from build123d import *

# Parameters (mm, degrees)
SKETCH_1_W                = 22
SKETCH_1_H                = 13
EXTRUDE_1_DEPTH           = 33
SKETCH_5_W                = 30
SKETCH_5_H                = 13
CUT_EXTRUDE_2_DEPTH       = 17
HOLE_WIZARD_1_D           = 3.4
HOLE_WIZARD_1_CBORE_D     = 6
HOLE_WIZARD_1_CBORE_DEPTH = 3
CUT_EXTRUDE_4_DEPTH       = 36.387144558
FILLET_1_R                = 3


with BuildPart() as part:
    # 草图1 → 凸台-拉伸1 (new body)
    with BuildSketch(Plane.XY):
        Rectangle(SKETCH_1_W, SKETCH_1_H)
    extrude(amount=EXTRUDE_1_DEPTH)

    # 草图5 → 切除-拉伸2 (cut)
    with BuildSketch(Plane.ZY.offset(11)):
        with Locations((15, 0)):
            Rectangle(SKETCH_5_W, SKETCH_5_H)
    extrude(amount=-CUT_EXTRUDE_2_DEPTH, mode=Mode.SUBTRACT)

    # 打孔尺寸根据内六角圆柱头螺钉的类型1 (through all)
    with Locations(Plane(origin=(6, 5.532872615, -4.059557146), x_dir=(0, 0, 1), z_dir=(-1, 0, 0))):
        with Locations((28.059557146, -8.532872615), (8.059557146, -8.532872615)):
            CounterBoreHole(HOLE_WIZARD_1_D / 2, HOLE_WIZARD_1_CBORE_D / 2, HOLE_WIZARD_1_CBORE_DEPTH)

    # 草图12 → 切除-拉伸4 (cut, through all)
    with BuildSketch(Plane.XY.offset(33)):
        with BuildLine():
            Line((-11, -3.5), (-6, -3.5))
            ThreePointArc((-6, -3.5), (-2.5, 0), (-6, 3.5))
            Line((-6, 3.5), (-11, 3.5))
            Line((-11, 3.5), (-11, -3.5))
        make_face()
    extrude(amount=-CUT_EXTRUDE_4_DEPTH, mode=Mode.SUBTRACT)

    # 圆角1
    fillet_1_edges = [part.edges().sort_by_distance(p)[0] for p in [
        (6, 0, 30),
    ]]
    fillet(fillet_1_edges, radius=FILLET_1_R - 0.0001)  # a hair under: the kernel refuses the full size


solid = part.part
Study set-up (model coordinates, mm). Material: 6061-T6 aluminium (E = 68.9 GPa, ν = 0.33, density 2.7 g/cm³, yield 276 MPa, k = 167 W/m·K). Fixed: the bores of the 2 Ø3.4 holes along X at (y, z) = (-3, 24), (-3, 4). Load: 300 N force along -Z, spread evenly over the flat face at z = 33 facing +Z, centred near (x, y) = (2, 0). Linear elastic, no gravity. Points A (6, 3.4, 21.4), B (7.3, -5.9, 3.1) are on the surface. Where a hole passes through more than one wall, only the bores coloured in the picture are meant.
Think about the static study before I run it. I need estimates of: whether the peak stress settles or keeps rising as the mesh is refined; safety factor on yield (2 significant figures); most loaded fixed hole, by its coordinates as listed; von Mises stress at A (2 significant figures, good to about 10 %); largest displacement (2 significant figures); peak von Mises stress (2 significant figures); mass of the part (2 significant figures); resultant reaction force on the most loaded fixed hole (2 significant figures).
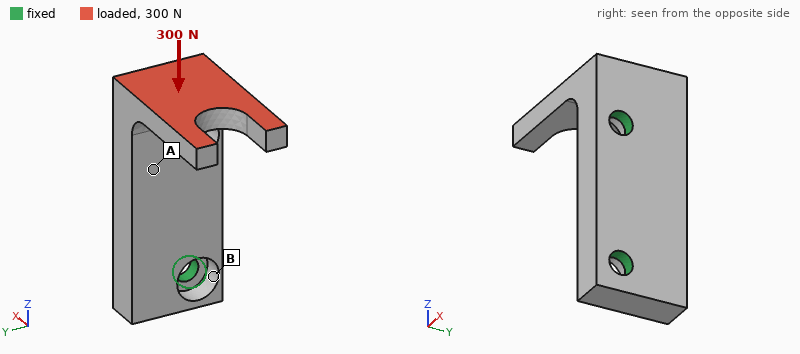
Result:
settles
1.6
(-3, 4)
34 MPa
0.11 mm
170 MPa
6.7 g
230 N
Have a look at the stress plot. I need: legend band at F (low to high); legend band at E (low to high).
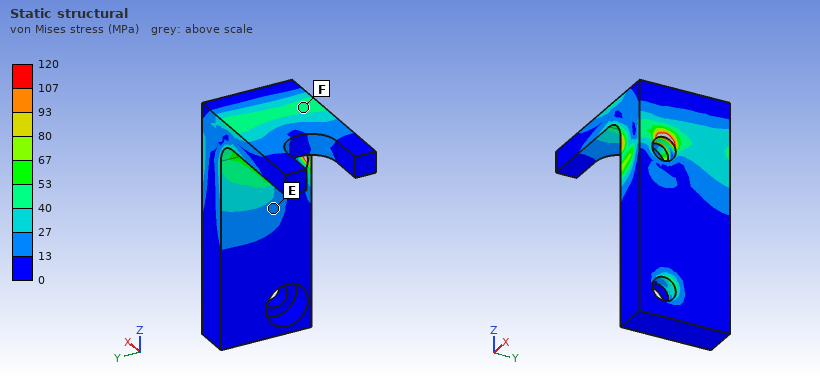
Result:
40 to 53 MPa
13 to 27 MPa
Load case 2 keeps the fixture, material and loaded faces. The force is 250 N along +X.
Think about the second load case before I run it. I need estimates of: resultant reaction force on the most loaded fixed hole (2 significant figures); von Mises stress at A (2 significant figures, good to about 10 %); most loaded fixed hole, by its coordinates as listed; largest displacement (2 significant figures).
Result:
340 N
29 MPa
(-3, 24)
67 µm
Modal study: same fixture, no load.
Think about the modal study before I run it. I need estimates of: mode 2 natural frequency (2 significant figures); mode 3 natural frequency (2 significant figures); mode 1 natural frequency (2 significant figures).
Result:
8300 Hz
15 kHz
7300 Hz
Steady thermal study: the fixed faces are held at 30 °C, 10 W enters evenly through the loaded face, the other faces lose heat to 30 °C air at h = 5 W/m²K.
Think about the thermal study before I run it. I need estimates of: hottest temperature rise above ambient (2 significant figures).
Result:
20 K
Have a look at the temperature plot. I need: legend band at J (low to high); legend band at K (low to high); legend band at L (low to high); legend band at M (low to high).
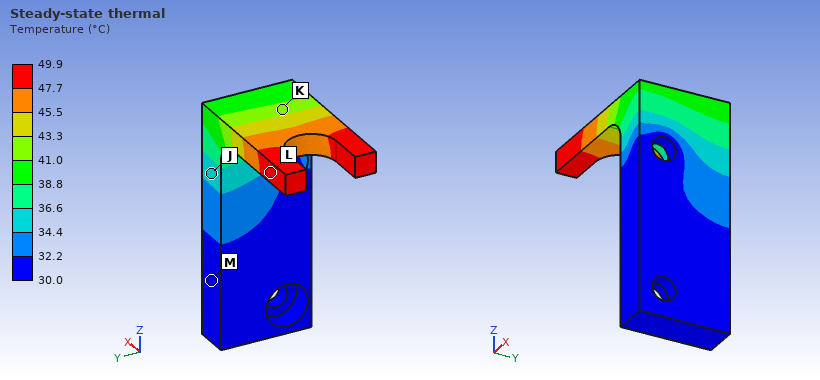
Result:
34.4 to 36.6 °C
41.0 to 43.3 °C
47.7 to 49.9 °C
30.0 to 32.2 °C
